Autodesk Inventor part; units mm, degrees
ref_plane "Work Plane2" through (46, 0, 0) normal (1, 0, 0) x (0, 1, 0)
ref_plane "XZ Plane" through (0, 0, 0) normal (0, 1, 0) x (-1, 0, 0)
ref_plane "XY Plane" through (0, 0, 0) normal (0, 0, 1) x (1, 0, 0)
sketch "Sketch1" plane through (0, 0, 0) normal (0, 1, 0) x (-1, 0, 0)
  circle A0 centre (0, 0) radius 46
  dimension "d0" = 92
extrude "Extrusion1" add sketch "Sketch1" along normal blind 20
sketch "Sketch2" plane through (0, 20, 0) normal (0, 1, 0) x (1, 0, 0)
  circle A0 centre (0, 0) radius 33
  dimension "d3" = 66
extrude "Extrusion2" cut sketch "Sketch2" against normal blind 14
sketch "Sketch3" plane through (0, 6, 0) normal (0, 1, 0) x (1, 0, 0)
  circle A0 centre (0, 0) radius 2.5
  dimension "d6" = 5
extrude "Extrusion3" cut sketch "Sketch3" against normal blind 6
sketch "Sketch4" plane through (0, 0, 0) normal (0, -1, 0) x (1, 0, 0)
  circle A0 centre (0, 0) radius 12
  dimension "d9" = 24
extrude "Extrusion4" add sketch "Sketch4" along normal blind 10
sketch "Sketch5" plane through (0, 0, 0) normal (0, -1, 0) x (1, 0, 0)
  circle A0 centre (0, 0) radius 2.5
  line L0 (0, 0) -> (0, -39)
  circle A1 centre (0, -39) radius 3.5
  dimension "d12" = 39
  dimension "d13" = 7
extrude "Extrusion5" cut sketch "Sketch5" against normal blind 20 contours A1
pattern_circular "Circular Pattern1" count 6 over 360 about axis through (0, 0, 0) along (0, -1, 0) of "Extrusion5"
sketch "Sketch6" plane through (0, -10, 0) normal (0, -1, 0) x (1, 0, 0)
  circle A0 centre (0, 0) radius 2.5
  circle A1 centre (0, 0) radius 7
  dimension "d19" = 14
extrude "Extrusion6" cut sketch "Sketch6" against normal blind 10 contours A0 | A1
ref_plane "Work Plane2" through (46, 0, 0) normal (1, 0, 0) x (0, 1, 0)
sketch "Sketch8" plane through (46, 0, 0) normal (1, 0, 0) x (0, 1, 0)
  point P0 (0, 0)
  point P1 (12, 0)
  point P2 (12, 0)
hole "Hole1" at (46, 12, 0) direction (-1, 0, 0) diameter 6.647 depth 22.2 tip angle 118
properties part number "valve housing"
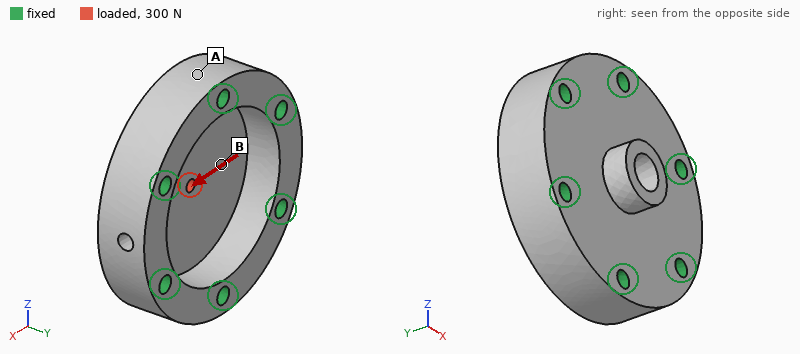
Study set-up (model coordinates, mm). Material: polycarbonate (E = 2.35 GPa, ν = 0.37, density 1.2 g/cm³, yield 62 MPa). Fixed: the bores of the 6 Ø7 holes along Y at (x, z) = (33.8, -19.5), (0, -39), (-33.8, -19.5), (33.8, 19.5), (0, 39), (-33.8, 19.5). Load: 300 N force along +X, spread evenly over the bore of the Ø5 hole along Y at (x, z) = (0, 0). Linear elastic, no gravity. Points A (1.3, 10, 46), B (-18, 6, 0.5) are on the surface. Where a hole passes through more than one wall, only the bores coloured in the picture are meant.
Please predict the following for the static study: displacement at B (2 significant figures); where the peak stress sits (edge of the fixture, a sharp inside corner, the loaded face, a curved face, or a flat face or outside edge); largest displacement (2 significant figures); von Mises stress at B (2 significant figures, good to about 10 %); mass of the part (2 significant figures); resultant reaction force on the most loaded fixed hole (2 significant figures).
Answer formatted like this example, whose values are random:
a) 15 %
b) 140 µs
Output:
a) 6.2 µm
b) the loaded face
c) 17 µm
d) 0.76 MPa
e) 99 g
f) 69 N
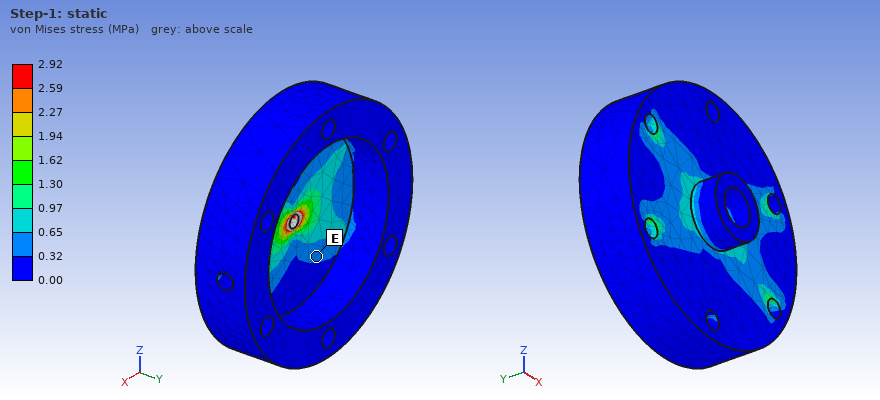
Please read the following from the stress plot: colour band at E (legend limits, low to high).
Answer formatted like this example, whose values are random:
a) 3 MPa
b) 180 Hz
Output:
a) 0.32 to 0.65 MPa
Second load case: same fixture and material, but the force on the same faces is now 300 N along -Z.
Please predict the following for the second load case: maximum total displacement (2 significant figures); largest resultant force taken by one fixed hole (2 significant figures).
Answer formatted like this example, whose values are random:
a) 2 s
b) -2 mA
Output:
a) 17 µm
b) 78 N
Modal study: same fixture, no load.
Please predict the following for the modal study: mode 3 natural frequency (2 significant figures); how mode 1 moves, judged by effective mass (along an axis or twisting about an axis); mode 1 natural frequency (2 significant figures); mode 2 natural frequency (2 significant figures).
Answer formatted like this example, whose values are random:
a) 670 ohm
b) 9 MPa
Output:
a) 5000 Hz
b) along Y
c) 2800 Hz
d) 4900 Hz
